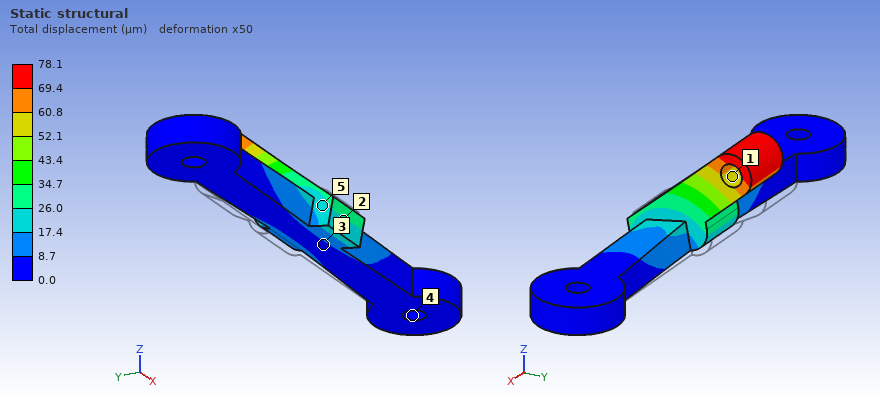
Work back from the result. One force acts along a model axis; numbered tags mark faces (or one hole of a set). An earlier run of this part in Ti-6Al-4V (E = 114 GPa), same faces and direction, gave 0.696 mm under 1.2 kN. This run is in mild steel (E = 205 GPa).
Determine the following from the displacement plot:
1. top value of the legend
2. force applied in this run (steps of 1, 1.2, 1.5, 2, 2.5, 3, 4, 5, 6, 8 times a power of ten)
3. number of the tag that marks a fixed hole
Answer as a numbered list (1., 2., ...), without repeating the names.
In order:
1. 78.1 µm
2. 250 N
3. 4
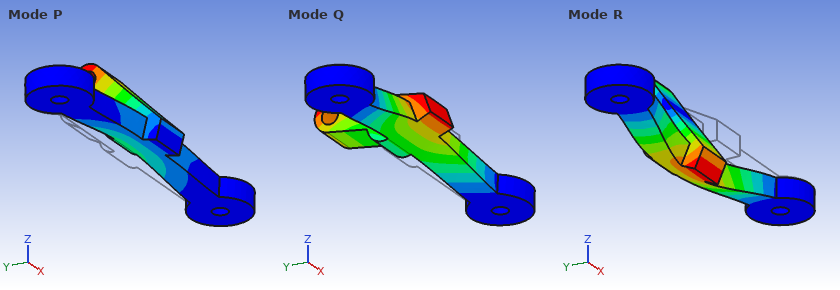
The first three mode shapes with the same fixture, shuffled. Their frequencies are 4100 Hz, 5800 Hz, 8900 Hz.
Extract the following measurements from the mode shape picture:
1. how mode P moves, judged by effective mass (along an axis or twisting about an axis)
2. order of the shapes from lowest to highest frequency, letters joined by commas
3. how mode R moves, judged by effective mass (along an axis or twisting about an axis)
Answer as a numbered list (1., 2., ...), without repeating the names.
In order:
1. along Z
2. P, Q, R
3. along Y
